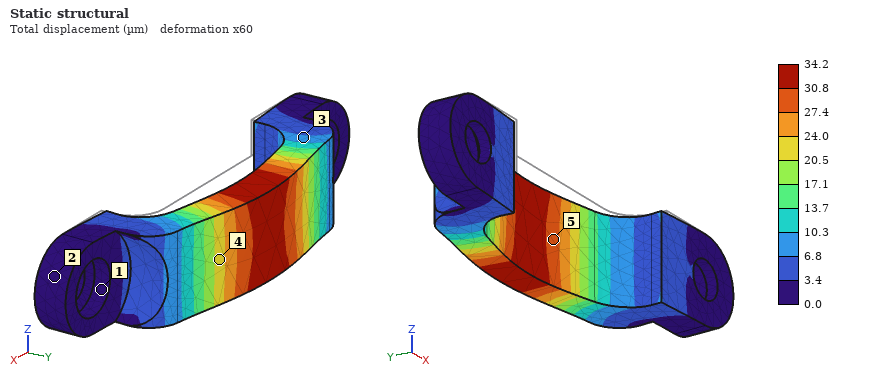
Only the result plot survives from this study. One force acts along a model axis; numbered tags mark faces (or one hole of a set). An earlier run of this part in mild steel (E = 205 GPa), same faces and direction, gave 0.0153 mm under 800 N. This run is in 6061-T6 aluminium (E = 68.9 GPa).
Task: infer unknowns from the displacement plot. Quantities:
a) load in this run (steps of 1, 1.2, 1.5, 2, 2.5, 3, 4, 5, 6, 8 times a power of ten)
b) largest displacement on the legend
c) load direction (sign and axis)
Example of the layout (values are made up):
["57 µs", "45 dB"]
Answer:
["600 N", "34.2 µm", "+Y"]
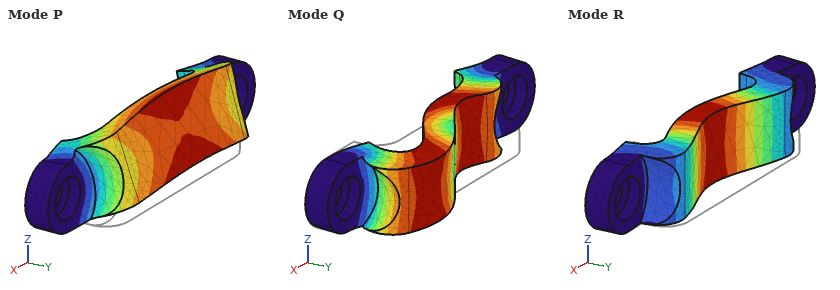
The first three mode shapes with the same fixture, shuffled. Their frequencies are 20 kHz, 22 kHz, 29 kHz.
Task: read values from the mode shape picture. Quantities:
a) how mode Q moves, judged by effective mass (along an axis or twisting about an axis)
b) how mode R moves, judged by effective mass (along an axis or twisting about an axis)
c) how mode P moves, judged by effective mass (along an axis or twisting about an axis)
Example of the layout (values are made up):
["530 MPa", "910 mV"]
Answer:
["along X", "along Y", "along Z"]
